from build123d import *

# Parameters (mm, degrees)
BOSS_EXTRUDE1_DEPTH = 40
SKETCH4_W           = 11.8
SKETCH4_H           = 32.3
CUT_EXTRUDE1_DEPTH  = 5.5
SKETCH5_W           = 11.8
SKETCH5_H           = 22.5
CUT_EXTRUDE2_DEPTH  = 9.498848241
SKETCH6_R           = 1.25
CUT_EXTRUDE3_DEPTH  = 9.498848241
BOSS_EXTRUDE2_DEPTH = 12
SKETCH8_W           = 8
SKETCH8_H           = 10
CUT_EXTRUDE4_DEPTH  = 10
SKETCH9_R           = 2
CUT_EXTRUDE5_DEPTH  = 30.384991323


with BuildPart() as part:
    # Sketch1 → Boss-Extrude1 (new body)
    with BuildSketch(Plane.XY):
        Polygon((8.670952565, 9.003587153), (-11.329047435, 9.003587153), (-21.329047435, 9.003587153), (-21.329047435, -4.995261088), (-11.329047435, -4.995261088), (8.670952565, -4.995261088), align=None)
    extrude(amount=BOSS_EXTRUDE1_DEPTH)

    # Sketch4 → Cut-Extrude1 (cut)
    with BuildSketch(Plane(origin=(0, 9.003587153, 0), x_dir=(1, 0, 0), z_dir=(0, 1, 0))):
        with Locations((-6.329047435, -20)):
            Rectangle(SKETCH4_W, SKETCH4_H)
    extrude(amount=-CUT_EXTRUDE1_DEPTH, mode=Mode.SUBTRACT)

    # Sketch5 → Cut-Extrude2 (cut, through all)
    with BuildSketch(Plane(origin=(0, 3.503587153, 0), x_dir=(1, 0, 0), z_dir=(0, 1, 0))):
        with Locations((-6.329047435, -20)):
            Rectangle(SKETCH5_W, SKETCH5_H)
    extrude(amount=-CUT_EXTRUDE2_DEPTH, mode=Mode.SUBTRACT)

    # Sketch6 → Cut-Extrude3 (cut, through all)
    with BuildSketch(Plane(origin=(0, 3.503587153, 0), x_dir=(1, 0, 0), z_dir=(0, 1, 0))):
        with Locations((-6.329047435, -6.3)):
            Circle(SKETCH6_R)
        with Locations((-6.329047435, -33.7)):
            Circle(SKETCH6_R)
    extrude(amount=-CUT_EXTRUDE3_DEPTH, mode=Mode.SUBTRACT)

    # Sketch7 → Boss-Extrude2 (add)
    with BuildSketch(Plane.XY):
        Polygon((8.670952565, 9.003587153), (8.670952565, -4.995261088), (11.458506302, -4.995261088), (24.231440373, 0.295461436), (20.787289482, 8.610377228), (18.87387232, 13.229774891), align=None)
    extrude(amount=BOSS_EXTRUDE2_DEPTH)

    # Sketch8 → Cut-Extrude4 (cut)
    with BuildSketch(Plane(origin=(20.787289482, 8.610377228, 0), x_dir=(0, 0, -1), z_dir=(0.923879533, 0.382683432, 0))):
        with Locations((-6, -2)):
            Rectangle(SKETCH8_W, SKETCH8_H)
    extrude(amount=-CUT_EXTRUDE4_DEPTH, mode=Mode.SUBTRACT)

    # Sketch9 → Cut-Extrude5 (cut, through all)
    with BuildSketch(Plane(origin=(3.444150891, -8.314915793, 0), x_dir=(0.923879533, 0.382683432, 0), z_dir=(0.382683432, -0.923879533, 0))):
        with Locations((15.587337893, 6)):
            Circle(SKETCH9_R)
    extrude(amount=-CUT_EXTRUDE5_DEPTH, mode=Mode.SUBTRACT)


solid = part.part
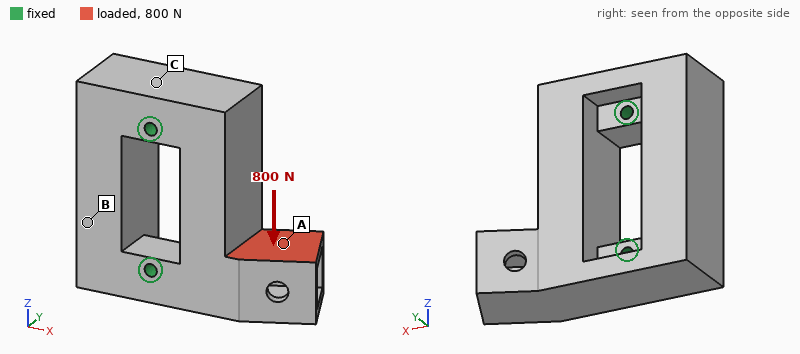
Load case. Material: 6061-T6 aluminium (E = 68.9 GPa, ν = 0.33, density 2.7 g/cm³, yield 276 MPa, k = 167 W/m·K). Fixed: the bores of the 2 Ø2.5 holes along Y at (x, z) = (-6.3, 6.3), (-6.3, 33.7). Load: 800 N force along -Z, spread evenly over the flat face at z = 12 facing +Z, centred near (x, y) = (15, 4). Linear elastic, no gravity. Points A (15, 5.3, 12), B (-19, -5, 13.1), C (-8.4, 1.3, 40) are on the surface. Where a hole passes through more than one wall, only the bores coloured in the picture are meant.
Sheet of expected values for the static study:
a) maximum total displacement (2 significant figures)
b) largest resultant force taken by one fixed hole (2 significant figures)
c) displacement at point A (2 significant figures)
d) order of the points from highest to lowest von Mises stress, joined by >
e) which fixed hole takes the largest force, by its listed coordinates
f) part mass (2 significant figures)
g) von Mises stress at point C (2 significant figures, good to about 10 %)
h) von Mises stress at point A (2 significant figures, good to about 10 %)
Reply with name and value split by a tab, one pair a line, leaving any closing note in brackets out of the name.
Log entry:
maximum total displacement	39 µm
largest resultant force taken by one fixed hole	790 N
displacement at point A	24 µm
order of the points from highest to lowest von Mises stress, joined by >	A > C > B
which fixed hole takes the largest force, by its listed coordinates	(-6.3, 33.7)
part mass	37 g
von Mises stress at point C	9.4 MPa
von Mises stress at point A	17 MPa
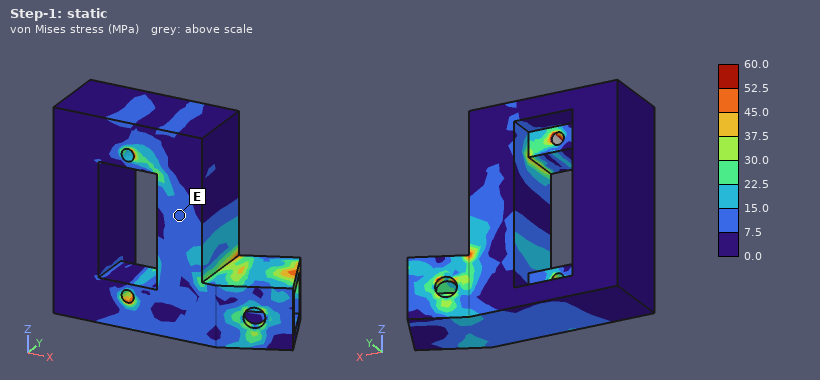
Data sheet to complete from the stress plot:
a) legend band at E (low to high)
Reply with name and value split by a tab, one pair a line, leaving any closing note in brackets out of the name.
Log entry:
legend band at E	7.5 to 15.0 MPa
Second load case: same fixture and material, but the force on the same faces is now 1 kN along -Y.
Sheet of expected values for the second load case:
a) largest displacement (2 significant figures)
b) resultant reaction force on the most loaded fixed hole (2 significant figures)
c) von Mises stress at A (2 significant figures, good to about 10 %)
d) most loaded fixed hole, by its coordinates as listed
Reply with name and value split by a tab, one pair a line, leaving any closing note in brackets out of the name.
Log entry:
largest displacement	89 µm
resultant reaction force on the most loaded fixed hole	750 N
von Mises stress at A	31 MPa
most loaded fixed hole, by its coordinates as listed	(-6.3, 6.3)
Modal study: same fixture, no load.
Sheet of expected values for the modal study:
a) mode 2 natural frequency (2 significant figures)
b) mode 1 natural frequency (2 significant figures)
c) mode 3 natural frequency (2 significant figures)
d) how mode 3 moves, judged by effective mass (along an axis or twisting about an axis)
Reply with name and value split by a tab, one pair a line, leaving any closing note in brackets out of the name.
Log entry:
mode 2 natural frequency	13 kHz
mode 1 natural frequency	8200 Hz
mode 3 natural frequency	14 kHz
how mode 3 moves, judged by effective mass	along Y
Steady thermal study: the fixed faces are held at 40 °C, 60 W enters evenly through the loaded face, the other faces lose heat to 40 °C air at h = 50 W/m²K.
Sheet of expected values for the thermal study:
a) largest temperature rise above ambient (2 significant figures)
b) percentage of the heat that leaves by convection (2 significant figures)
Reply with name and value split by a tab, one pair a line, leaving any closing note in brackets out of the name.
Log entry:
largest temperature rise above ambient	78 K
percentage of the heat that leaves by convection	7.8 %
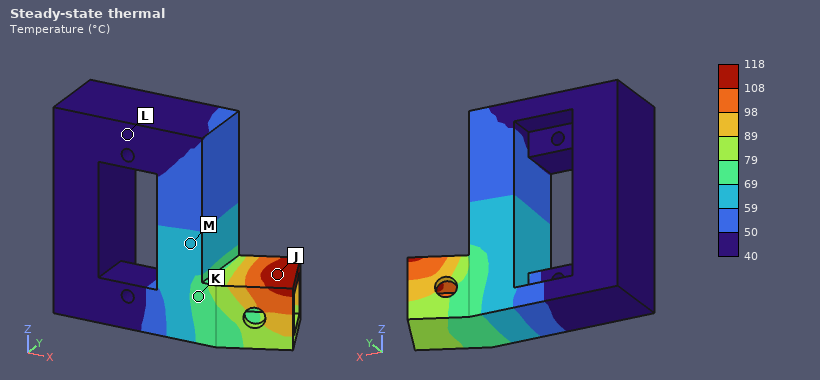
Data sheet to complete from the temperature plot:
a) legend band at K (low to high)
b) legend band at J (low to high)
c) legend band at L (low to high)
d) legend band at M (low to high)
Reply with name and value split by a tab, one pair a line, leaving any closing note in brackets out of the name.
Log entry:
legend band at K	69 to 79 °C
legend band at J	108 to 118 °C
legend band at L	40 to 50 °C
legend band at M	59 to 69 °C
